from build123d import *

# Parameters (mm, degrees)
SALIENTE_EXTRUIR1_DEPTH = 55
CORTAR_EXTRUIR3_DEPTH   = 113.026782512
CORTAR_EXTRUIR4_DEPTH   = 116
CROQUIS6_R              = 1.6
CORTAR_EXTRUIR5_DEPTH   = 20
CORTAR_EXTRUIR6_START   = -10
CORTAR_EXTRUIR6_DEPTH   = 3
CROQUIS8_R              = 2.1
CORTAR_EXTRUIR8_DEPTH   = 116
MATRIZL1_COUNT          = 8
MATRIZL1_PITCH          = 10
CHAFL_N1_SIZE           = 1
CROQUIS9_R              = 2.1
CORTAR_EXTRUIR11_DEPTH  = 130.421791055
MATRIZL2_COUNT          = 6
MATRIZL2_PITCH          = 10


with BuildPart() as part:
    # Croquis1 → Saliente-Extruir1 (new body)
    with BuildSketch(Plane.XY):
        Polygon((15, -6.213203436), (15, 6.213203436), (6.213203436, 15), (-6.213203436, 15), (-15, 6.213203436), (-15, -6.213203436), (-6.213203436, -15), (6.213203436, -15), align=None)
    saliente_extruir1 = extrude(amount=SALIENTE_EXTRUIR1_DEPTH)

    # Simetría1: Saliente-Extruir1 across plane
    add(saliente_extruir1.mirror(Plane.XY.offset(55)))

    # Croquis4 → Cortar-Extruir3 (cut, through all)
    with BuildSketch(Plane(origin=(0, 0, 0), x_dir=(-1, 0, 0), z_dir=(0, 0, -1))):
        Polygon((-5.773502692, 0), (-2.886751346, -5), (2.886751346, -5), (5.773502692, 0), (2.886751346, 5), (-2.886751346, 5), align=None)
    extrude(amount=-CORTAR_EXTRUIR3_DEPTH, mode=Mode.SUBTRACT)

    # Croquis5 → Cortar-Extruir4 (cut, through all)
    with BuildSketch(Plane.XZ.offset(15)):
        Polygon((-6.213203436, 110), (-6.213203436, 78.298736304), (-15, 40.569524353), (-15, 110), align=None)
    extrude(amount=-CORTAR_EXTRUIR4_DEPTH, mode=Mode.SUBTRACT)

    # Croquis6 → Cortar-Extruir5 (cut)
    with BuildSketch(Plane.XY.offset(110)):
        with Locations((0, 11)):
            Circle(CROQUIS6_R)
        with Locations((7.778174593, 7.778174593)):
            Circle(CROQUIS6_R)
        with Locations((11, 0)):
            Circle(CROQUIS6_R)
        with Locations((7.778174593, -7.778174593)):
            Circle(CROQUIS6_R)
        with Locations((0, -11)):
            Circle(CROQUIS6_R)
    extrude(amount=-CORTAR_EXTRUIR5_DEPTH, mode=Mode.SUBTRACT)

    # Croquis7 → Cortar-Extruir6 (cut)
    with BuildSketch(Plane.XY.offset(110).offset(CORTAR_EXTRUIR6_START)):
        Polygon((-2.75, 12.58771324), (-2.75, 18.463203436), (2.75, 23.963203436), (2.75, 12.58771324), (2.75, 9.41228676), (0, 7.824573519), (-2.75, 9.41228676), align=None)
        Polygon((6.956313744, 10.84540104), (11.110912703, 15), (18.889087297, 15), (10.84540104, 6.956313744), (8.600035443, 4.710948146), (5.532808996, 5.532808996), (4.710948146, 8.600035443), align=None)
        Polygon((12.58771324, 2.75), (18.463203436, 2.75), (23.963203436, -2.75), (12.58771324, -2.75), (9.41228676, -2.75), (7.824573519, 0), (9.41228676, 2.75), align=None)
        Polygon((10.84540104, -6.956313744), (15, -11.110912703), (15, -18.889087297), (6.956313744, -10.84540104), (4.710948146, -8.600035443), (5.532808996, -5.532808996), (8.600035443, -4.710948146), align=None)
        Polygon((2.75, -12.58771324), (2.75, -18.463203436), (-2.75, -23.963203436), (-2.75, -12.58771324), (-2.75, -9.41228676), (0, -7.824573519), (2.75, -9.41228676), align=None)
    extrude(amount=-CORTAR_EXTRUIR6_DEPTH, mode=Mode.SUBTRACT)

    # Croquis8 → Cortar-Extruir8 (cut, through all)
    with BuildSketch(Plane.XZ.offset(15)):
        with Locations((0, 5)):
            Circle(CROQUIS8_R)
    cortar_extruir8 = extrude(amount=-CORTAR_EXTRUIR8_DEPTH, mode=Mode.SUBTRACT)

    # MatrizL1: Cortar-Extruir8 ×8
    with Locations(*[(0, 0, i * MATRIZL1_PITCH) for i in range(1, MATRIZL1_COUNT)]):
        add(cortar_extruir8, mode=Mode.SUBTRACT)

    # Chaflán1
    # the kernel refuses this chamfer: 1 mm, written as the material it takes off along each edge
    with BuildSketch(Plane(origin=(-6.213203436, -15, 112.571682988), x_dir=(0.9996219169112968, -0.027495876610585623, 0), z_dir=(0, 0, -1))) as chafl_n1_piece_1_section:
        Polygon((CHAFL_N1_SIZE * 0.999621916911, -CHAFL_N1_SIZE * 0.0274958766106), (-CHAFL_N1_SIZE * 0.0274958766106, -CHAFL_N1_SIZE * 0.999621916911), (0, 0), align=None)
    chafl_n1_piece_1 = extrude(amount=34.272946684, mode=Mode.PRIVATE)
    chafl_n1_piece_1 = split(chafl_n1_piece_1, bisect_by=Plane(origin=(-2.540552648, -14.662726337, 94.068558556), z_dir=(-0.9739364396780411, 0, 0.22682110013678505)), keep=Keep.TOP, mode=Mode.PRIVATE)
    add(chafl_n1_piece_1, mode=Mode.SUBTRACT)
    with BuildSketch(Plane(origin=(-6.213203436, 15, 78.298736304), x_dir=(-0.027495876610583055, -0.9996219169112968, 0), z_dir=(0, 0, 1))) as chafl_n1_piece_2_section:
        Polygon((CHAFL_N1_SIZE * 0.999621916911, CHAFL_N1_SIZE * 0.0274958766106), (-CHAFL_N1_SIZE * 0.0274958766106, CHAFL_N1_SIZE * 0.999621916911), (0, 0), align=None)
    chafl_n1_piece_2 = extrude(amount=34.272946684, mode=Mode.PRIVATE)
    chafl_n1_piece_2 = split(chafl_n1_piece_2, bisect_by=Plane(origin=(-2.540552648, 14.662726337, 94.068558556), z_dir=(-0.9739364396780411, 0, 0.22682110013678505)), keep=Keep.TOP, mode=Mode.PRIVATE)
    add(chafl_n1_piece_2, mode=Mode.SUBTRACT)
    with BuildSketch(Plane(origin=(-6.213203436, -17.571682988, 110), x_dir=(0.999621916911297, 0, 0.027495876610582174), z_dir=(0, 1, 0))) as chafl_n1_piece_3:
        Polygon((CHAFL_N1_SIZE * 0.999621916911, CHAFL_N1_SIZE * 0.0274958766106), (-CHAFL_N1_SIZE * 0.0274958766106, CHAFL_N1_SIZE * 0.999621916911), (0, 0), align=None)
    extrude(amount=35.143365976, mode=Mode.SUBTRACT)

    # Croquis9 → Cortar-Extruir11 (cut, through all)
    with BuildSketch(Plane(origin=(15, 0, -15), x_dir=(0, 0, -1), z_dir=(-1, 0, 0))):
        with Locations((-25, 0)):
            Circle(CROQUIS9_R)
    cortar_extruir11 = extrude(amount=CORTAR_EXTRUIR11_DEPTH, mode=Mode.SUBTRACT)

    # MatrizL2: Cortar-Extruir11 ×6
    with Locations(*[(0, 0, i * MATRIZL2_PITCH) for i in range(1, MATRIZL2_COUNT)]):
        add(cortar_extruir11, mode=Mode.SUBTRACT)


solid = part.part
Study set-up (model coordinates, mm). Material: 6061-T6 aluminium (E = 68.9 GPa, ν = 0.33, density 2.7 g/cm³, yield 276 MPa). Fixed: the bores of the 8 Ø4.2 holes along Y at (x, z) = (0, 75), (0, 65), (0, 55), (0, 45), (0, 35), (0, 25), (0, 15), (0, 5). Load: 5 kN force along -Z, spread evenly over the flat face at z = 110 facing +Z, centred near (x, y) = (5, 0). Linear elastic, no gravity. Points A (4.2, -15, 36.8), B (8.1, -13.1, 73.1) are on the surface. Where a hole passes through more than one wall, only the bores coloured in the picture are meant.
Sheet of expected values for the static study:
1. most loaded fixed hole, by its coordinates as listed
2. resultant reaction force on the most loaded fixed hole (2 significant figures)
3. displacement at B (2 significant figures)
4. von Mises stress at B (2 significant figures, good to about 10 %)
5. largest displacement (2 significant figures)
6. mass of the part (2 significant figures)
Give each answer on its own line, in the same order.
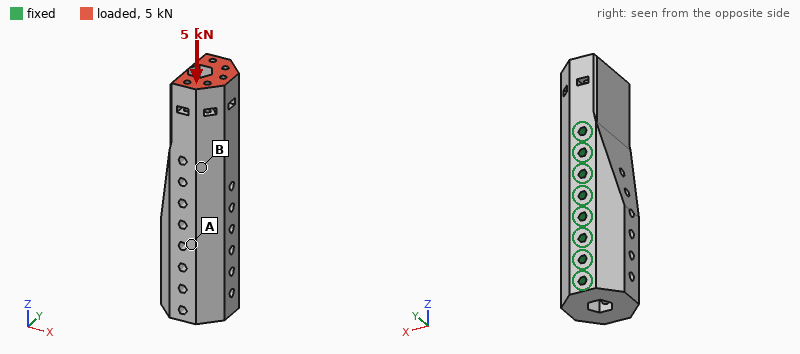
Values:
(0, 75)
2.2 kN
7.0 µm
13 MPa
20 µm
160 g
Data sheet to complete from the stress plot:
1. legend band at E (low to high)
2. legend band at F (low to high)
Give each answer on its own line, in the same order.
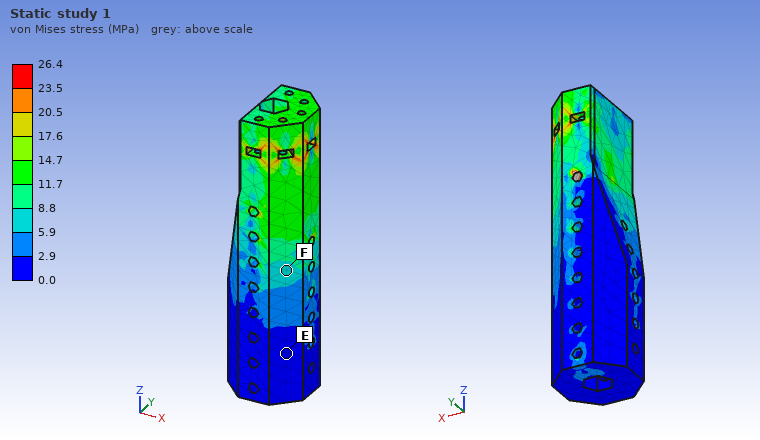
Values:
0.0 to 2.9 MPa
5.9 to 8.8 MPa
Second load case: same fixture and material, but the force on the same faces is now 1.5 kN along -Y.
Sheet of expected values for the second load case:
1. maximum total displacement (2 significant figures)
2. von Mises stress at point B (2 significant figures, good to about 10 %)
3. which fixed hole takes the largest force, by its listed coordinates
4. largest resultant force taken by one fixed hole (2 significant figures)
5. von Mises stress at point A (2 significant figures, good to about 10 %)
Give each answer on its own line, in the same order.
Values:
36 µm
16 MPa
(0, 75)
2.5 kN
3.9 MPa
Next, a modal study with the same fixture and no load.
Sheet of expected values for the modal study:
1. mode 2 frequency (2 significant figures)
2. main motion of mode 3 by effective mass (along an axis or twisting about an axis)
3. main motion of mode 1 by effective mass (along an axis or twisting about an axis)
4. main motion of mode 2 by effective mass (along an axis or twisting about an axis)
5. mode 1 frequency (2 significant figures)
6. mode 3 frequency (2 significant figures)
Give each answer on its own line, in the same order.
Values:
9000 Hz
along X
along X
along Y
6900 Hz
11 kHz
